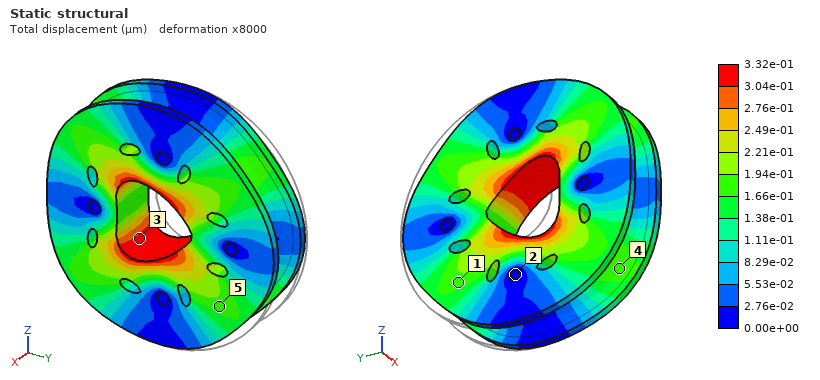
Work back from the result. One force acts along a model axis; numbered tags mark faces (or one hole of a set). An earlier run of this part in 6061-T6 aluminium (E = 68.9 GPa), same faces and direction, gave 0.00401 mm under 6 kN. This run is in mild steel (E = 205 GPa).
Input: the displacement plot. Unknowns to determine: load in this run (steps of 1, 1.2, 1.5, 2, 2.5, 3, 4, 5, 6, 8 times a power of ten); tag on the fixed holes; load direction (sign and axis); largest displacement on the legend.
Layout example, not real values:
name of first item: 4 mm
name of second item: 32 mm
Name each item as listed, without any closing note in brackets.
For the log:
load in this run: 1.5 kN
tag on the fixed holes: 2
load direction: -Y
largest displacement on the legend: 3.32e-01 µm
